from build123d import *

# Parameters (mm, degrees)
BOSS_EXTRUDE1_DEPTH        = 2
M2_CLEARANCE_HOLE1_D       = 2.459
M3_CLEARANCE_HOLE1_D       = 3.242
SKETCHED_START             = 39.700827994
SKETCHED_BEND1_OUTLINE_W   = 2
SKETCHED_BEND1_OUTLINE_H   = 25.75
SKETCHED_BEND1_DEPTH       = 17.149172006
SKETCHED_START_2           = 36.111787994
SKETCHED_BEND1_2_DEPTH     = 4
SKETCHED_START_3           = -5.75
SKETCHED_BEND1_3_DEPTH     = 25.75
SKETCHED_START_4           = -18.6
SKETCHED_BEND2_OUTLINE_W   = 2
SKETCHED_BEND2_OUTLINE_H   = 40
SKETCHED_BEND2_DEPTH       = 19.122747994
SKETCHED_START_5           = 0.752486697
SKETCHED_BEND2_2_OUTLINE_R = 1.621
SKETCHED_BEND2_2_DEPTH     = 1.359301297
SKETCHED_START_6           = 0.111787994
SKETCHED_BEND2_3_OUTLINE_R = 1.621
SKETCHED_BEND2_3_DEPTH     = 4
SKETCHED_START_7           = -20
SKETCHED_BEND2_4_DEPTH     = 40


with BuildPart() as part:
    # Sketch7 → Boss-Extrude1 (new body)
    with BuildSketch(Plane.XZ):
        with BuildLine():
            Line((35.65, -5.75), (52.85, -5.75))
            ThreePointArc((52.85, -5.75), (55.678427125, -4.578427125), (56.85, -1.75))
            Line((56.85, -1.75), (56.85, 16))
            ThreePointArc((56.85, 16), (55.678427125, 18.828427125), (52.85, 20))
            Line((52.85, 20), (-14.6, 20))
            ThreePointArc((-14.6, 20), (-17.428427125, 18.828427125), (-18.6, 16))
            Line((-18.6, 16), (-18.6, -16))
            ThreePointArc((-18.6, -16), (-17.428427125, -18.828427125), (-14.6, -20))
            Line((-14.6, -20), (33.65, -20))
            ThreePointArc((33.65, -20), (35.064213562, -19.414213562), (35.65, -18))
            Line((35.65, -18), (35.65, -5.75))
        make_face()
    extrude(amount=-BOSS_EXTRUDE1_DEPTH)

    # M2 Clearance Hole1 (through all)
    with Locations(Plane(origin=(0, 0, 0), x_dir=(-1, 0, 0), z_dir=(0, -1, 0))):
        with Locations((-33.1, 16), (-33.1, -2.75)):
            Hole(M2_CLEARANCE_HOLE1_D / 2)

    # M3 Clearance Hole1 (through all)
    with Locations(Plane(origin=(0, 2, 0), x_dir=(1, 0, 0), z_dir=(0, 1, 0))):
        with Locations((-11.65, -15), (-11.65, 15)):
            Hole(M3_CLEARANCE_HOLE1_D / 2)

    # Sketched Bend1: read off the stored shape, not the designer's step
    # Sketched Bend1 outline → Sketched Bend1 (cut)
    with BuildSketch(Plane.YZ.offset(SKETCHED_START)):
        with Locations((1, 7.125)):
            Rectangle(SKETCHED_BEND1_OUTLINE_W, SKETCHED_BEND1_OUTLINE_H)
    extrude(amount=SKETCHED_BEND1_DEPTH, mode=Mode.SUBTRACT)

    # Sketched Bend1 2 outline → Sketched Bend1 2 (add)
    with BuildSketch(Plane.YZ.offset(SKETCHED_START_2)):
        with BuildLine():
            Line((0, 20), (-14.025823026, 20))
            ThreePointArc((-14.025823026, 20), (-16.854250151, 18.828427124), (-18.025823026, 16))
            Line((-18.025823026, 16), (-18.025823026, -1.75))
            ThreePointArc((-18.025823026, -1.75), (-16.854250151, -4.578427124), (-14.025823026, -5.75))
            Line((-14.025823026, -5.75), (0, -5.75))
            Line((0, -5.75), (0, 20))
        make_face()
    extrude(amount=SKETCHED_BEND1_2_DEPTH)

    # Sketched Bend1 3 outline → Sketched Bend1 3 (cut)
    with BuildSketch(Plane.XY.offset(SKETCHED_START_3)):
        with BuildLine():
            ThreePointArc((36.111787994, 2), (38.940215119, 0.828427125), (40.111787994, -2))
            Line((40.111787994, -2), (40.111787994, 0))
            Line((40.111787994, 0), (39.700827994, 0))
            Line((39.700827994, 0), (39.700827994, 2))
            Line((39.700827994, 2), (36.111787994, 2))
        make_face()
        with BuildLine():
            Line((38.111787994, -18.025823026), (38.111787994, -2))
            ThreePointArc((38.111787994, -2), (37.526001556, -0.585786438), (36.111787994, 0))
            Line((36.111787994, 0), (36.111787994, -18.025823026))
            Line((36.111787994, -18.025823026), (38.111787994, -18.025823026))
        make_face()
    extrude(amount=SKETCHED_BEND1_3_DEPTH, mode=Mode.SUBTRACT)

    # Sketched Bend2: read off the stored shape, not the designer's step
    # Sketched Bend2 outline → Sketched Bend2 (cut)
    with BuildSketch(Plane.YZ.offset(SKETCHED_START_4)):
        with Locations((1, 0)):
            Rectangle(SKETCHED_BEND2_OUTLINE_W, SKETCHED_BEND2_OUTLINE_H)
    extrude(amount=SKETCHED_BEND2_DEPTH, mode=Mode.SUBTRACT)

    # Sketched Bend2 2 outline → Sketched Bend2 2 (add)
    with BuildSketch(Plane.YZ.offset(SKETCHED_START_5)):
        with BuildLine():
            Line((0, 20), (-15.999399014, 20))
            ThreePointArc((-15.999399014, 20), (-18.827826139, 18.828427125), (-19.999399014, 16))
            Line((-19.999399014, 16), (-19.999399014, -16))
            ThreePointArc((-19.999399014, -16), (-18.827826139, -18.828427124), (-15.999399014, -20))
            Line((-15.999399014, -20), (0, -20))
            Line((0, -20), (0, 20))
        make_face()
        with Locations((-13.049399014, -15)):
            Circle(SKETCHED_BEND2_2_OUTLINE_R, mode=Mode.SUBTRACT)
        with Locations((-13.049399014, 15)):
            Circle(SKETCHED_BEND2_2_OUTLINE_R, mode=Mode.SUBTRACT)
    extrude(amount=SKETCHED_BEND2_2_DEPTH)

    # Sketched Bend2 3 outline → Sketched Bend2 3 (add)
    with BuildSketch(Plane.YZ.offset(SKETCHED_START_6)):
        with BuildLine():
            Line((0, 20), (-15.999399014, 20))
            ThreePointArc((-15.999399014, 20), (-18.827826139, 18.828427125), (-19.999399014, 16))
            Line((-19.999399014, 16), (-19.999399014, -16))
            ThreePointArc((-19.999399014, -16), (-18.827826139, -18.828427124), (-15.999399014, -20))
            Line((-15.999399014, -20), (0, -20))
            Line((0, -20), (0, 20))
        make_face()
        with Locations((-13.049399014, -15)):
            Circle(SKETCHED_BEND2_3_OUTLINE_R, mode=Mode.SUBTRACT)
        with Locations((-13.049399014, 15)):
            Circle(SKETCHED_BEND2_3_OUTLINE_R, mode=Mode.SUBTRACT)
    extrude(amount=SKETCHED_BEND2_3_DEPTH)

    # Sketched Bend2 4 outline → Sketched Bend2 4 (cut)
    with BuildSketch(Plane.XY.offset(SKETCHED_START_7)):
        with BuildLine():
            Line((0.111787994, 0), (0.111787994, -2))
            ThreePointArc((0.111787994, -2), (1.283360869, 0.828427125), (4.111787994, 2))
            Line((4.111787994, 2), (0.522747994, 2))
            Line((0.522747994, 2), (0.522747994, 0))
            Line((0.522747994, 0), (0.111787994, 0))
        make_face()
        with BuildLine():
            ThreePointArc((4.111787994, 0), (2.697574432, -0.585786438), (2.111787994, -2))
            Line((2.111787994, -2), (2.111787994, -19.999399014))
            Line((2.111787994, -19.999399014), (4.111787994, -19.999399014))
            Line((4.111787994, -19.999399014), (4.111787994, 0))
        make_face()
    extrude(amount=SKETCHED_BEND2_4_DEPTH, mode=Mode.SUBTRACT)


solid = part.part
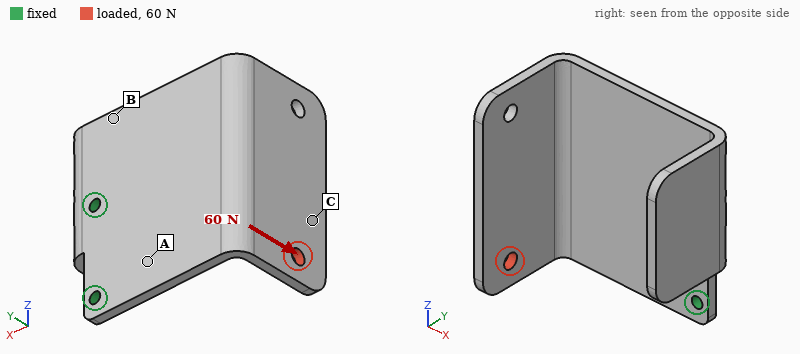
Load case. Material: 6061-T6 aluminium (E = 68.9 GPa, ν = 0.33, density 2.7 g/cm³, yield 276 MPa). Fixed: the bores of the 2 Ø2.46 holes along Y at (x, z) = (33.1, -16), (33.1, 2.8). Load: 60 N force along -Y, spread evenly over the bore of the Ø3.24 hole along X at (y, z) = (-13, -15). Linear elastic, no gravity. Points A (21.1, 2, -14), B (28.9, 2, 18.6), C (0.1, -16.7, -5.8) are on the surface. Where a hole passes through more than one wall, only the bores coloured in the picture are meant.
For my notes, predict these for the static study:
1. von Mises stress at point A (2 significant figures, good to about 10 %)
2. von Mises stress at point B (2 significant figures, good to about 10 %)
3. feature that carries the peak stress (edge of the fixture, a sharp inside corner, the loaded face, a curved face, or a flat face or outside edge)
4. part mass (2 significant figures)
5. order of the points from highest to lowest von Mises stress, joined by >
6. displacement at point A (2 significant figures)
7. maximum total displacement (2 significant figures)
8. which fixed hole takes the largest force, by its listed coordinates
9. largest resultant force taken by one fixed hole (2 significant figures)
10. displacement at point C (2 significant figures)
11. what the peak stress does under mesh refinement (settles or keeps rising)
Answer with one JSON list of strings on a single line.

["55 MPa", "30 MPa", "edge of the fixture", "14 g", "A > B > C", "0.095 mm", "0.63 mm", "(33.1, -16)", "56 N", "0.53 mm", "keeps rising"]
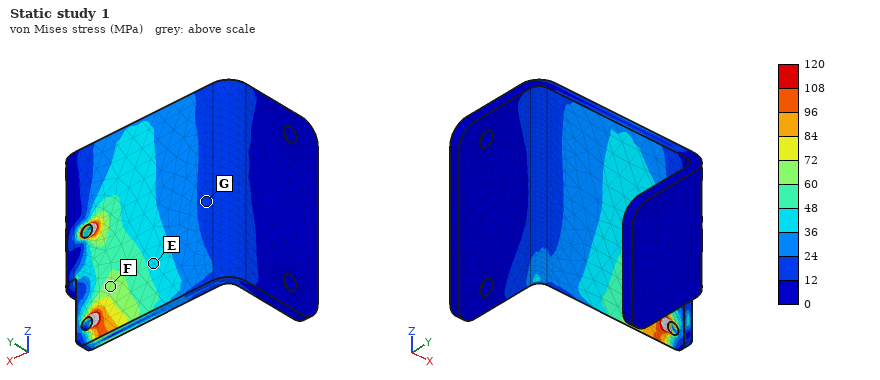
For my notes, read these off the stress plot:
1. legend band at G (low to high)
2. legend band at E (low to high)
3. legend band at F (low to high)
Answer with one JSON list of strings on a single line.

["12 to 24 MPa", "36 to 48 MPa", "60 to 72 MPa"]
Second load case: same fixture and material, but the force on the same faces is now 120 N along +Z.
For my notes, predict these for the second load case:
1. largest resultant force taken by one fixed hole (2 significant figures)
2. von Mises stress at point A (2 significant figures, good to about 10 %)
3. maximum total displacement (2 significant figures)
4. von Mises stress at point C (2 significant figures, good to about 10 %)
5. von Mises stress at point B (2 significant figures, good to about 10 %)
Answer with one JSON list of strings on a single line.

["210 N", "43 MPa", "0.40 mm", "9.6 MPa", "33 MPa"]
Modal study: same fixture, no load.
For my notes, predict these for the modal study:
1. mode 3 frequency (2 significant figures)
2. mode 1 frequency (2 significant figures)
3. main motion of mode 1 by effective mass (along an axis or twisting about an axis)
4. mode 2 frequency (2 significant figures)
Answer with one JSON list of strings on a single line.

["2600 Hz", "730 Hz", "along Y", "1500 Hz"]
